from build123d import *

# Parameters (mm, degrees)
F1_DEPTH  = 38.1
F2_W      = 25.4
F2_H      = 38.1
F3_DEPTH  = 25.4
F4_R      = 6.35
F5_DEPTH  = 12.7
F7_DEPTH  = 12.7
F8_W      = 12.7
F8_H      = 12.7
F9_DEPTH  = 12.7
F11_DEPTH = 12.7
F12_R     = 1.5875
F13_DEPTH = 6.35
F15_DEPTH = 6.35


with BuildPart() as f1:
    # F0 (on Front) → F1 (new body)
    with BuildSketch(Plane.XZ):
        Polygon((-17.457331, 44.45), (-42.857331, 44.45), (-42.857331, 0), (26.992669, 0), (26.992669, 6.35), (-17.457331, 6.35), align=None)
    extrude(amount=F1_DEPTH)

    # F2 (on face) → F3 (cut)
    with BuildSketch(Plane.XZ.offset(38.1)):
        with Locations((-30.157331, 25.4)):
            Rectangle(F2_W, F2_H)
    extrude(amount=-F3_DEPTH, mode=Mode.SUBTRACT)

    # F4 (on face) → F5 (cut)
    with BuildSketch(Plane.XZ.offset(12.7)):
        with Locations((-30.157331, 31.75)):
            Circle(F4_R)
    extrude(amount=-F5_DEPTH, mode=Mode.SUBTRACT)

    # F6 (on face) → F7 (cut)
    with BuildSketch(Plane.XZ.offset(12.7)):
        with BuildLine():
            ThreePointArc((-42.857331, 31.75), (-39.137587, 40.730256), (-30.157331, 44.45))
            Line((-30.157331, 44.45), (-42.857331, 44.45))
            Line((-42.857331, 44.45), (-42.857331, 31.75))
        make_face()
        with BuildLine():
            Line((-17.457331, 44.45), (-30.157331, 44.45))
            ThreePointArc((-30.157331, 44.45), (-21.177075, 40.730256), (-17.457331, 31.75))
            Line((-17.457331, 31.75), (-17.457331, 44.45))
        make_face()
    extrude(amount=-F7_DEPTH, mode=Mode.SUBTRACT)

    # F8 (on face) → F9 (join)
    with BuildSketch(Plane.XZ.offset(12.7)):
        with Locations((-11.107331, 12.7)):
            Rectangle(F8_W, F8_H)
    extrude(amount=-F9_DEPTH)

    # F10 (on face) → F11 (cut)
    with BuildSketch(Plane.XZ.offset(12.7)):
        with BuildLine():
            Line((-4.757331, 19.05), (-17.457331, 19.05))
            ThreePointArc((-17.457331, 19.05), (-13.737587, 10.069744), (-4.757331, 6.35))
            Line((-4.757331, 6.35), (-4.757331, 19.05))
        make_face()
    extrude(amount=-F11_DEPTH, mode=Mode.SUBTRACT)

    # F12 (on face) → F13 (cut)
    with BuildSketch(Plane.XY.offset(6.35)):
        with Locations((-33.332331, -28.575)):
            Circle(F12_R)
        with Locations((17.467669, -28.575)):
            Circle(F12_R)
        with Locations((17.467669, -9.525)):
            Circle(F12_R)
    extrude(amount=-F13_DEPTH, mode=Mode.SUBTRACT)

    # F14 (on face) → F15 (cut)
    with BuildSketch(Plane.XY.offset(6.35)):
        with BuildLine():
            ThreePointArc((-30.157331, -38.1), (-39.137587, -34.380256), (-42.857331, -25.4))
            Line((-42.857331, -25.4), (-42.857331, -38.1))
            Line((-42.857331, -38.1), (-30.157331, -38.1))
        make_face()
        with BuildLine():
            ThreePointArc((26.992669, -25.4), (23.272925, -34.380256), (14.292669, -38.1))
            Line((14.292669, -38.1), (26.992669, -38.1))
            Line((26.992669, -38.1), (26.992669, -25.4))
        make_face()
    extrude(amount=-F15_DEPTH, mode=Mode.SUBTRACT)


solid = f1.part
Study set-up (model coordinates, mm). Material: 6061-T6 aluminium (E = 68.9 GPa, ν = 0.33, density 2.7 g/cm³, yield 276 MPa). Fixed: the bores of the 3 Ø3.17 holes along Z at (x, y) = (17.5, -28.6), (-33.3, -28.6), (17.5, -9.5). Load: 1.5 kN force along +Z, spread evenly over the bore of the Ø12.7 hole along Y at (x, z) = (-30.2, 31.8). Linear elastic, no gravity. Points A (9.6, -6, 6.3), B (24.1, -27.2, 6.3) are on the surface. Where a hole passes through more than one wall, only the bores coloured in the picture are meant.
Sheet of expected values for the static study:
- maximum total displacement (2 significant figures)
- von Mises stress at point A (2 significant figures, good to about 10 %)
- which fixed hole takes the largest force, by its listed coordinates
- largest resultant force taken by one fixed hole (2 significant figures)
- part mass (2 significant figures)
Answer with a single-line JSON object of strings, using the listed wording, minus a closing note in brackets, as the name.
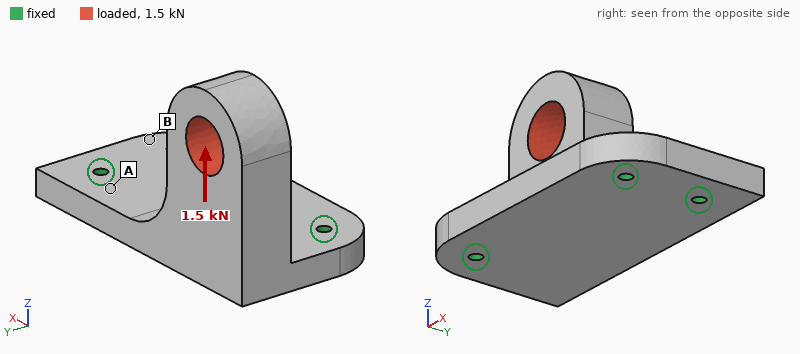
{"maximum total displacement": "0.27 mm", "von Mises stress at point A": "42 MPa", "which fixed hole takes the largest force, by its listed coordinates": "(-33.3, -28.6)", "largest resultant force taken by one fixed hole": "1.3 kN", "part mass": "72 g"}
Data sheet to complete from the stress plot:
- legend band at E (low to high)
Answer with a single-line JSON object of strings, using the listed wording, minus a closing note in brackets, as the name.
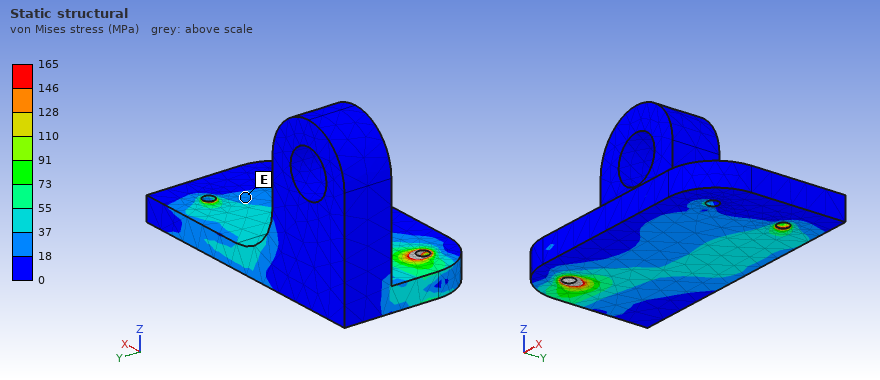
{"legend band at E": "18 to 37 MPa"}
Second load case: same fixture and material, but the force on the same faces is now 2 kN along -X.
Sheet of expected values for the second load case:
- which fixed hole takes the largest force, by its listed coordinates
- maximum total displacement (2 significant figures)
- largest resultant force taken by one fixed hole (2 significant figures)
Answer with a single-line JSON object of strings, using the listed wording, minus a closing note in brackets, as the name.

{"which fixed hole takes the largest force, by its listed coordinates": "(-33.3, -28.6)", "maximum total displacement": "0.27 mm", "largest resultant force taken by one fixed hole": "1.4 kN"}
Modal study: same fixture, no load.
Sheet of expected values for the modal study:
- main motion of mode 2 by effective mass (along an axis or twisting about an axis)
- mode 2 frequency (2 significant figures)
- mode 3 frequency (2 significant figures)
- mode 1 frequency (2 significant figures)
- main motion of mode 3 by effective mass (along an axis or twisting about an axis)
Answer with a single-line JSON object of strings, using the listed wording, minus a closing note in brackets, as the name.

{"main motion of mode 2 by effective mass": "along X", "mode 2 frequency": "4300 Hz", "mode 3 frequency": "6300 Hz", "mode 1 frequency": "2100 Hz", "main motion of mode 3 by effective mass": "along Z"}
